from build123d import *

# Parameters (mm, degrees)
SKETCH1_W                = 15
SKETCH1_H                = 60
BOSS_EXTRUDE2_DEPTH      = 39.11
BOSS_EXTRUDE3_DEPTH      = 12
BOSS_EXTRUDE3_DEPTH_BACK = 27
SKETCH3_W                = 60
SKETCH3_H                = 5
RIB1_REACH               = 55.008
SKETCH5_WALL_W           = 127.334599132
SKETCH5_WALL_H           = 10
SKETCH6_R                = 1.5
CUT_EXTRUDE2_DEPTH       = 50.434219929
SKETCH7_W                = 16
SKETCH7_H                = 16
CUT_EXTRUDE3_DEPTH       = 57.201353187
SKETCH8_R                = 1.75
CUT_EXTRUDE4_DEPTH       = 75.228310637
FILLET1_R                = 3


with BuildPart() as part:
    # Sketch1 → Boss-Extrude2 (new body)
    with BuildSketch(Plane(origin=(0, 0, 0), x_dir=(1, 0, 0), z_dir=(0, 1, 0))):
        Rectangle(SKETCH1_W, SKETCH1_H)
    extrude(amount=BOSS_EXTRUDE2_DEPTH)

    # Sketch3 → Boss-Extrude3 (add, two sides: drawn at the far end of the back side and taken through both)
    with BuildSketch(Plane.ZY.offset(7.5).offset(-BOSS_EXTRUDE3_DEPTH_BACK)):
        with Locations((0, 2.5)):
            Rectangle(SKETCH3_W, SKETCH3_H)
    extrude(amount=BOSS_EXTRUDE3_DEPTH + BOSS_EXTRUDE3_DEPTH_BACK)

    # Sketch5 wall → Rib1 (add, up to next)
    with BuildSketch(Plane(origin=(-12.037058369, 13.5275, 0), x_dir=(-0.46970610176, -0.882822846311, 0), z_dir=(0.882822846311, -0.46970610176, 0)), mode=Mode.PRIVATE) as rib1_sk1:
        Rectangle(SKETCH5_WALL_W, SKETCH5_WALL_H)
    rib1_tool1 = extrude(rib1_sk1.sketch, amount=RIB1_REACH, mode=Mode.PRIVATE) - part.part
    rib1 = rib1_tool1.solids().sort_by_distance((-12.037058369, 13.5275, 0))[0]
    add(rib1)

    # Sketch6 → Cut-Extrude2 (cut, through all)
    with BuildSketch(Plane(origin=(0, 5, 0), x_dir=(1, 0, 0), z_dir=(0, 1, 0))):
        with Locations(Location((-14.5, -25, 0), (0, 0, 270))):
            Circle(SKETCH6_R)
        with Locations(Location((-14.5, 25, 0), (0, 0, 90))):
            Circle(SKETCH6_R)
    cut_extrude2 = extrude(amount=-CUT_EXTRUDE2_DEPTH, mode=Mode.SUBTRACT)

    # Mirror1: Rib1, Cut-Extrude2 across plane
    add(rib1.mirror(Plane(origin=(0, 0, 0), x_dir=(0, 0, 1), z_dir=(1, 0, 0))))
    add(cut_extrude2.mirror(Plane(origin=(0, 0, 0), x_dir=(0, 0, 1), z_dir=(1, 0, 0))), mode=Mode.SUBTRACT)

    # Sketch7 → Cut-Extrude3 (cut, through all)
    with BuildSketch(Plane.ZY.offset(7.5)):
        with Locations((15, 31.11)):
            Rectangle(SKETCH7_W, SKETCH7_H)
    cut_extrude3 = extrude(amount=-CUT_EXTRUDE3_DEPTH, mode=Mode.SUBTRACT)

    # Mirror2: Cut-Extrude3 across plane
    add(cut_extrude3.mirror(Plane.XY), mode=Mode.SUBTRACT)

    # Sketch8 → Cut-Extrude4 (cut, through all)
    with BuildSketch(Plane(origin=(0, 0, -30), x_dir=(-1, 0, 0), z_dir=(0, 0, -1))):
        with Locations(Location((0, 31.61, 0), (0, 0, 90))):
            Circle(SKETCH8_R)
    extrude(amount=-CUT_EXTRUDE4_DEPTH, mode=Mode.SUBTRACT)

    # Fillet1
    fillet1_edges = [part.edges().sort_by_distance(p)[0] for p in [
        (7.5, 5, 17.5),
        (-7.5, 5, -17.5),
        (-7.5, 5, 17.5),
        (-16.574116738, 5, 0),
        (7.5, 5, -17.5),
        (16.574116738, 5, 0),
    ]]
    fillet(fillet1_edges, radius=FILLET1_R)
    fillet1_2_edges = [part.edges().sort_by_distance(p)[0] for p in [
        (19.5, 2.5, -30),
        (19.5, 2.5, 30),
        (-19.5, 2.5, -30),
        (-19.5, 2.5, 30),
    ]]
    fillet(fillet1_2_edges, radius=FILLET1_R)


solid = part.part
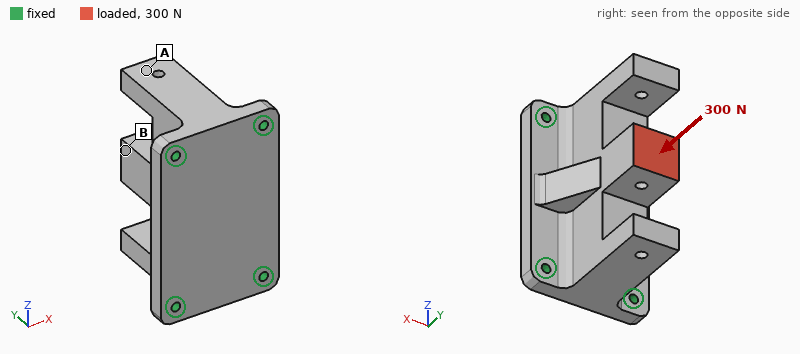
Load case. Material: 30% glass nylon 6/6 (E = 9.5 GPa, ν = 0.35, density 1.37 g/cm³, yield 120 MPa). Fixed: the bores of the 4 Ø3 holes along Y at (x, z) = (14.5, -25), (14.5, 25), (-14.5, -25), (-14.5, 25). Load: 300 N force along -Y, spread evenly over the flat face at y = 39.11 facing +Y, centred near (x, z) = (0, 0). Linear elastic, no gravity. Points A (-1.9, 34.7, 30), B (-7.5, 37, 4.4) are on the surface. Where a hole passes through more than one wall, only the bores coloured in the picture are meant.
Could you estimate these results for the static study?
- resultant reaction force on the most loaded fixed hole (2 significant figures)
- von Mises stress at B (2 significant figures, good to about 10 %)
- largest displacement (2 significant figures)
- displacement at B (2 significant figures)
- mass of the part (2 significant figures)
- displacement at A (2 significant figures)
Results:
87 N
1.4 MPa
13 µm
12 µm
49 g
5.9 µm
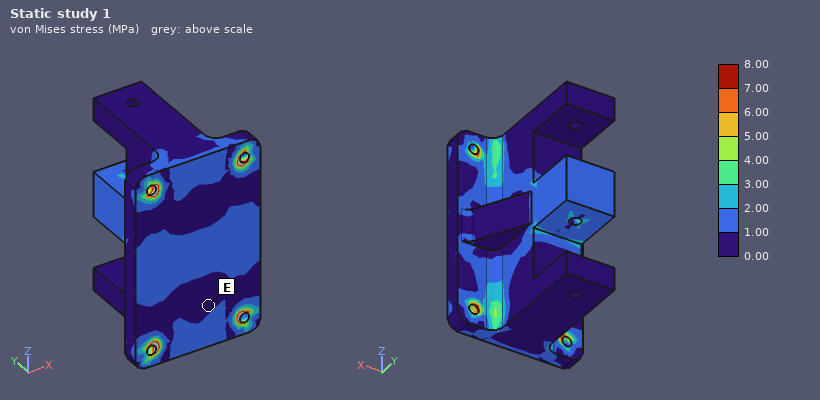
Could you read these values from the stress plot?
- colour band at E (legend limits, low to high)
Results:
0.00 to 1.00 MPa
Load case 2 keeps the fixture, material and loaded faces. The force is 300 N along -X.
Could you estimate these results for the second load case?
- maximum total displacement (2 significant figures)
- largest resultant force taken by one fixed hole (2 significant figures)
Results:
0.13 mm
230 N
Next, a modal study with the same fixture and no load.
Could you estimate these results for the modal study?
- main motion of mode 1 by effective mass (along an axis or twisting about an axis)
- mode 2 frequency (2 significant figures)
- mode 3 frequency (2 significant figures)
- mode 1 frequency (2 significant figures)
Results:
along X
4800 Hz
4900 Hz
3300 Hz
